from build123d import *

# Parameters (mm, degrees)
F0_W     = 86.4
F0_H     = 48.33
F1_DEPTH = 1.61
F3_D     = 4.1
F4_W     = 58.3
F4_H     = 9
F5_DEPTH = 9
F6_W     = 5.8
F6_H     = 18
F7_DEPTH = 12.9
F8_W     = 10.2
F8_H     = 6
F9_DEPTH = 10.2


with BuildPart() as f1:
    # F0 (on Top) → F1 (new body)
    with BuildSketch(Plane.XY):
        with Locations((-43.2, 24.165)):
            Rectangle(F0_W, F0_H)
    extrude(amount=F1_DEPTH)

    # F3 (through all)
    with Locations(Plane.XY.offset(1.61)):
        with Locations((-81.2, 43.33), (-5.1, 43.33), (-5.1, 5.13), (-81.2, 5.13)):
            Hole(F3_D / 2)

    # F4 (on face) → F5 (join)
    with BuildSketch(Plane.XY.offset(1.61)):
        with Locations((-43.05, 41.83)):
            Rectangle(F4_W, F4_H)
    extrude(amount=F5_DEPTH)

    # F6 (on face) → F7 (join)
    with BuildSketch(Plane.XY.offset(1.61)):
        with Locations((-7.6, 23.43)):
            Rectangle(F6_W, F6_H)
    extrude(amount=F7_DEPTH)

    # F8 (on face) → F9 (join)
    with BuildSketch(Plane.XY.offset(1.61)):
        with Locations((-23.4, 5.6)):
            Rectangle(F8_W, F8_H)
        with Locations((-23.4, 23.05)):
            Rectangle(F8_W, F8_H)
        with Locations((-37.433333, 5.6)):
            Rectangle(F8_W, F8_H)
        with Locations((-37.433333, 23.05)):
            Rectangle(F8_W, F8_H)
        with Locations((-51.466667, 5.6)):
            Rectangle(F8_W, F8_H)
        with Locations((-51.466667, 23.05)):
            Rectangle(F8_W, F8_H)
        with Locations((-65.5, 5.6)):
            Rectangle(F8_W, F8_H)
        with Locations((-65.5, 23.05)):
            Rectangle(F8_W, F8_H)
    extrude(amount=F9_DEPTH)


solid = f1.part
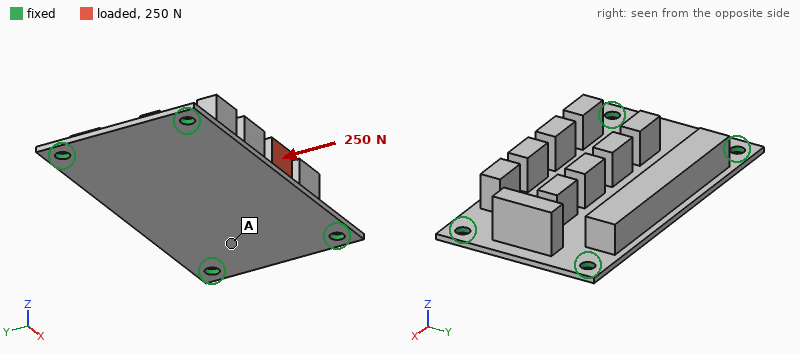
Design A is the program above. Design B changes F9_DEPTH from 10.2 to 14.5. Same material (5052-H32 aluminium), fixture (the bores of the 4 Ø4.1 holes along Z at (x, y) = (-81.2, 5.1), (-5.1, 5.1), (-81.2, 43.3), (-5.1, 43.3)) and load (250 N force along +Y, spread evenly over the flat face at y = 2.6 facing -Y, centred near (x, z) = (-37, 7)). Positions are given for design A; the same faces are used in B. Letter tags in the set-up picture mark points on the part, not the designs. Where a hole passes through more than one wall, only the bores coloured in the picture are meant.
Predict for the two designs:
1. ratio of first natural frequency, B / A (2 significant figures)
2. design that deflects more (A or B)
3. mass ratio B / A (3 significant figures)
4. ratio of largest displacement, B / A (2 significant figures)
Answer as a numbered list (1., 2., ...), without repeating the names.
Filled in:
1. 0.86
2. B
3. 1.12
4. 1.7
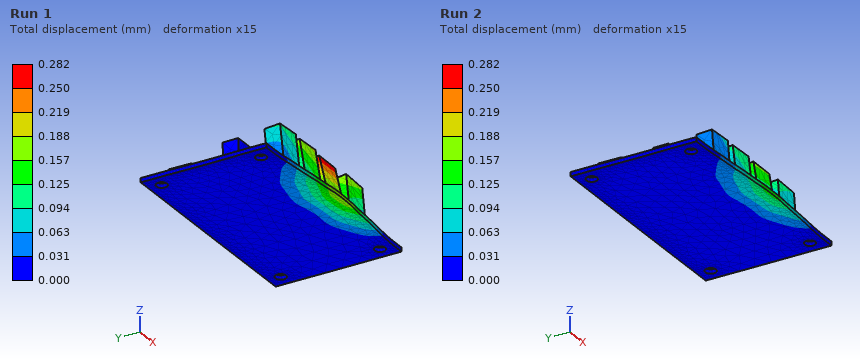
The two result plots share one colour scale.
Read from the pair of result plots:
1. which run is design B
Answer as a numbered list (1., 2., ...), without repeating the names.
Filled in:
1. Run 1
